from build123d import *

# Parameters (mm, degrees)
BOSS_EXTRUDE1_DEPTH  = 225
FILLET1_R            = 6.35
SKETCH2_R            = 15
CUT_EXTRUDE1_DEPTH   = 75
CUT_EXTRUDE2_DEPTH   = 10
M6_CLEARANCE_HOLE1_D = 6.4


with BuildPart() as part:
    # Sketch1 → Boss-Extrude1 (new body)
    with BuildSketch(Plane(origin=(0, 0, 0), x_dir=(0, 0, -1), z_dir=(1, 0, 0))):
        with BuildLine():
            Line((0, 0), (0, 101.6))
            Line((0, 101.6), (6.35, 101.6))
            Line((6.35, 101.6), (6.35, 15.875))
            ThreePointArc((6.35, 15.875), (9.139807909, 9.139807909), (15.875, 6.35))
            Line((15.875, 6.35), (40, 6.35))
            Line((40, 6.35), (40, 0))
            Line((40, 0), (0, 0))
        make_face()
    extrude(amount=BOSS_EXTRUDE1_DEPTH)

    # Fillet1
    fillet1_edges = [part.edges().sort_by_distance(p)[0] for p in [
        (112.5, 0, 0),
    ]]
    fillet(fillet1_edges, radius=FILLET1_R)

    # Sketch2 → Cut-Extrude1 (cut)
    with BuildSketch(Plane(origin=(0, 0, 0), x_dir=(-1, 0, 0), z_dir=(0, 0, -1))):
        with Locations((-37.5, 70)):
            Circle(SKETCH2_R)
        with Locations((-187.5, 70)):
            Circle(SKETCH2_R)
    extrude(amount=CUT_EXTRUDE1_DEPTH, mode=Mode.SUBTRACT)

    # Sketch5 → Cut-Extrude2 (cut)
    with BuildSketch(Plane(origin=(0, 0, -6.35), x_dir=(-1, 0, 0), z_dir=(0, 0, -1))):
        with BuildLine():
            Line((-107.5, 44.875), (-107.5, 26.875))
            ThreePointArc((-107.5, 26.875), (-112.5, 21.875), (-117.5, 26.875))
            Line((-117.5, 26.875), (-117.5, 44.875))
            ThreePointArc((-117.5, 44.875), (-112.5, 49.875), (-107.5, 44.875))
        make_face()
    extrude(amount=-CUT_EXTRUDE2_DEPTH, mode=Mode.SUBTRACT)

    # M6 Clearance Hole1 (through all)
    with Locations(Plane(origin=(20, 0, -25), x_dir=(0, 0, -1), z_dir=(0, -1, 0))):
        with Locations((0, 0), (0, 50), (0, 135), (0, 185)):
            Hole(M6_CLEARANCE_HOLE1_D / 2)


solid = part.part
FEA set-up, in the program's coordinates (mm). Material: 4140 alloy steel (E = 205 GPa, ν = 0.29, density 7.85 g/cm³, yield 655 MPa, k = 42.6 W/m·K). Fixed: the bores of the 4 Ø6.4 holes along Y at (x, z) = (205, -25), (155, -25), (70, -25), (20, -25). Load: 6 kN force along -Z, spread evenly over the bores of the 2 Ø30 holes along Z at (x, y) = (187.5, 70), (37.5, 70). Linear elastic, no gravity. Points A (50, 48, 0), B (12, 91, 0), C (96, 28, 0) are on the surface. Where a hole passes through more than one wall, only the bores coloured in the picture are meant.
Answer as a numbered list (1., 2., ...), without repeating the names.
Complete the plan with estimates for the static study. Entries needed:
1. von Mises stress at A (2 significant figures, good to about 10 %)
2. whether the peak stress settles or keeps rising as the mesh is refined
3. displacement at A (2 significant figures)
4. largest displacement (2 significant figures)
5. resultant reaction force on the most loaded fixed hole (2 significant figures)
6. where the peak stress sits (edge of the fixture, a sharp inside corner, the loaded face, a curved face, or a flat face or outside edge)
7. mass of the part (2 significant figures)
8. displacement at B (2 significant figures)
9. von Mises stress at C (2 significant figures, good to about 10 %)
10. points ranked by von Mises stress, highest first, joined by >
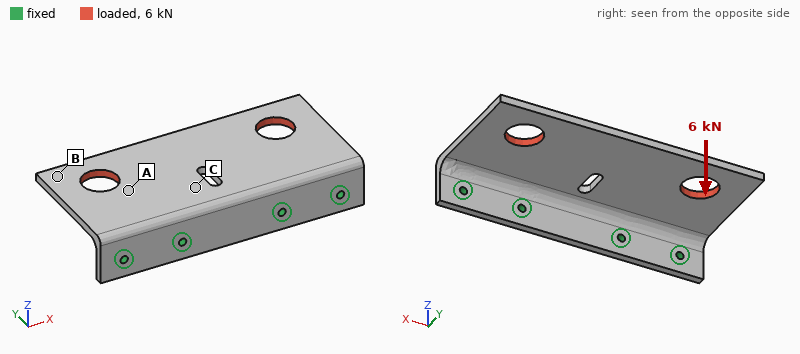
1. 84 MPa
2. keeps rising
3. 0.61 mm
4. 1.7 mm
5. 1.7 kN
6. edge of the fixture
7. 1.4 kg
8. 1.5 mm
9. 150 MPa
10. C > A > B
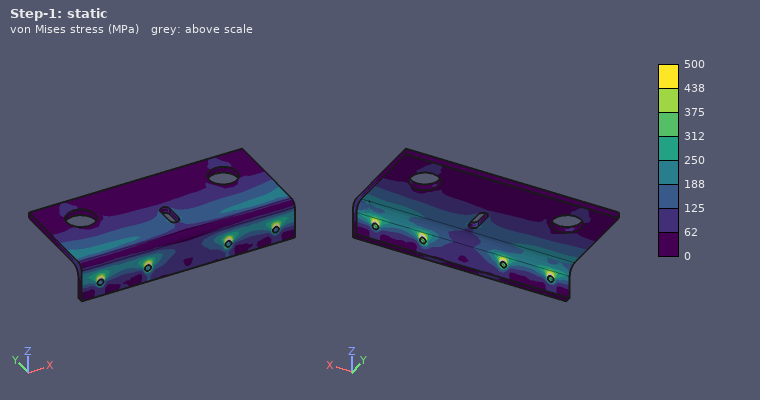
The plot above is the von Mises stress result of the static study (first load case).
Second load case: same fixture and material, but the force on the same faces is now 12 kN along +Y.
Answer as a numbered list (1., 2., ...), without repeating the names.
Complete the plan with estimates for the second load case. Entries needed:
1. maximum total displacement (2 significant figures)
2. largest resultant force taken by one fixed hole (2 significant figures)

1. 0.37 mm
2. 3.0 kN
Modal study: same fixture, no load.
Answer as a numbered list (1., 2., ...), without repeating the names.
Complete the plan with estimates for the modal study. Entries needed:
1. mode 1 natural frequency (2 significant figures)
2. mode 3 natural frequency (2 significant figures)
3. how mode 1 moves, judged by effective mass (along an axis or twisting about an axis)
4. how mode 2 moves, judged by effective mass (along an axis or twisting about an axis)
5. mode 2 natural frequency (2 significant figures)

1. 450 Hz
2. 1400 Hz
3. along Z
4. twisting about Y
5. 720 Hz
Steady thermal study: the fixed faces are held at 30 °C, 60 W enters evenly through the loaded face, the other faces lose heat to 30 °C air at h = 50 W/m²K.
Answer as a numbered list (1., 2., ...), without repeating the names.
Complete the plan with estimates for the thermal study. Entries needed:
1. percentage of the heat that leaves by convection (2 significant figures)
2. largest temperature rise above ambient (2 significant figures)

1. 78 %
2. 48 K
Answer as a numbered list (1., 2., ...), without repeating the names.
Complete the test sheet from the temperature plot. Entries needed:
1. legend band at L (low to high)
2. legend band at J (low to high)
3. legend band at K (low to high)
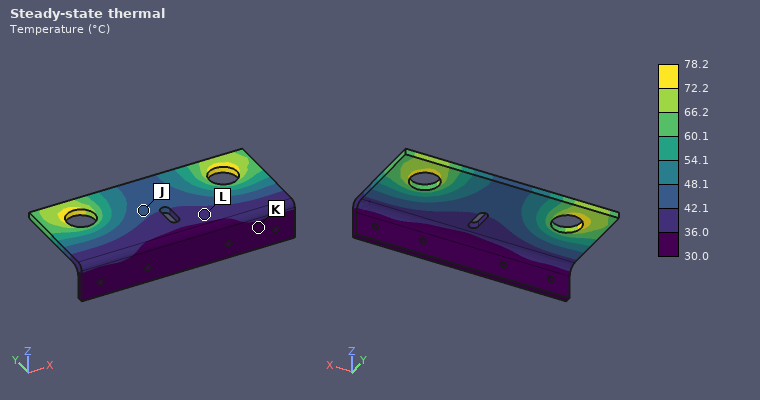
1. 36.0 to 42.1 °C
2. 42.1 to 48.1 °C
3. 30.0 to 36.0 °C
